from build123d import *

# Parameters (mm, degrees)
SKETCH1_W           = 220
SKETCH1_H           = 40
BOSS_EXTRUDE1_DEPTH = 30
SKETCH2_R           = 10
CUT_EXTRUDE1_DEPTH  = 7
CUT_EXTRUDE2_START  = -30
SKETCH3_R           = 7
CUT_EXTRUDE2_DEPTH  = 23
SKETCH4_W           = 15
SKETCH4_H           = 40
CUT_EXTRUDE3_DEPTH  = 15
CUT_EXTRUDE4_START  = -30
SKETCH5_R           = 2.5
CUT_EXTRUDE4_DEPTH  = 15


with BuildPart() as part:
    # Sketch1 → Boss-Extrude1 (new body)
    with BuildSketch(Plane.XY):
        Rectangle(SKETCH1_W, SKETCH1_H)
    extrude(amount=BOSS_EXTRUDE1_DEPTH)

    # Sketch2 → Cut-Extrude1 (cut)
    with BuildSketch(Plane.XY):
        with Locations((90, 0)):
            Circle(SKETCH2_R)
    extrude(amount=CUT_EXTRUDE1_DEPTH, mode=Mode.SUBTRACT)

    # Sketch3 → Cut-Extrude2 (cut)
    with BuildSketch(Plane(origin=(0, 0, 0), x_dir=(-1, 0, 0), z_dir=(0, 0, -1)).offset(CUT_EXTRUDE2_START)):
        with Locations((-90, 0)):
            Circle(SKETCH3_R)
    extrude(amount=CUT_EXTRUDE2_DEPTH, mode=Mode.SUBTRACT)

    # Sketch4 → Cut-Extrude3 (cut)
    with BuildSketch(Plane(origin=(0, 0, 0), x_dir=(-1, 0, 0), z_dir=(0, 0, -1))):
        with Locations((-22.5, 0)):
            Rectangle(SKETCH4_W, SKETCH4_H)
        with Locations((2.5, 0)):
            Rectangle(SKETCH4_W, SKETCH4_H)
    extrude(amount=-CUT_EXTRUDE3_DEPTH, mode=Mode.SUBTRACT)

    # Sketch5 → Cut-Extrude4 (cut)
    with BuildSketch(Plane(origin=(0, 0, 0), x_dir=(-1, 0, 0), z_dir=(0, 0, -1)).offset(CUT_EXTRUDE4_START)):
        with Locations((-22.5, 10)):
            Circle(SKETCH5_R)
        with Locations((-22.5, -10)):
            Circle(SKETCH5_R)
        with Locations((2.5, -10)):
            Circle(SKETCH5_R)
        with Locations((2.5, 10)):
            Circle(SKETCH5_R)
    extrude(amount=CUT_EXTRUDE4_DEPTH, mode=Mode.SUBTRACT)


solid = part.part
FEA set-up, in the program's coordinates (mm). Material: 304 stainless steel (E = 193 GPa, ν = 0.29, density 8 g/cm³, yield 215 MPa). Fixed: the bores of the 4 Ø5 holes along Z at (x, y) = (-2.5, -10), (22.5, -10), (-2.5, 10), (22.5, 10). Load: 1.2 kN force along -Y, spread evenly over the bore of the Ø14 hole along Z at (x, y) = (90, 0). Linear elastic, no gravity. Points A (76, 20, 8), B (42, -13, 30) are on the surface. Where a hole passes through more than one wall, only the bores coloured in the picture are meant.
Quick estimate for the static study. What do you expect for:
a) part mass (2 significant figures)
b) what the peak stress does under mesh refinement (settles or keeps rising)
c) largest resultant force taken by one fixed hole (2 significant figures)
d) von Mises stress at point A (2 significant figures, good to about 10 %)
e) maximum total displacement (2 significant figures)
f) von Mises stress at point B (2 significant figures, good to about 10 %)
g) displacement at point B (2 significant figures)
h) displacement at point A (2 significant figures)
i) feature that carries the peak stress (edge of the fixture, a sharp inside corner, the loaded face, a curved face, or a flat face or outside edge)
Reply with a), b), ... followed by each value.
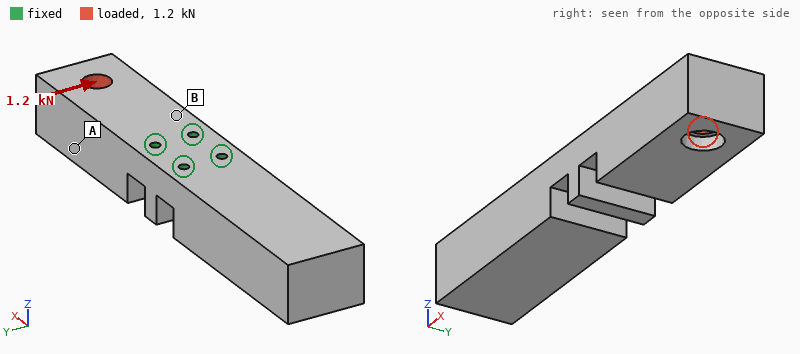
a) 1.9 kg
b) keeps rising
c) 2.9 kN
d) 2.5 MPa
e) 13 µm
f) 8.7 MPa
g) 2.3 µm
h) 7.3 µm
i) edge of the fixture
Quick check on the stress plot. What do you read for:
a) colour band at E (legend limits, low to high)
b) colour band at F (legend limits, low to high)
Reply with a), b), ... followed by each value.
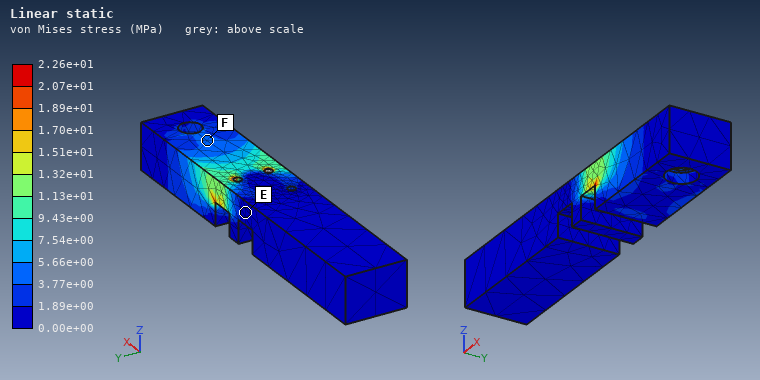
a) 0.00e+00 to 1.89e+00 MPa
b) 3.77e+00 to 5.66e+00 MPa
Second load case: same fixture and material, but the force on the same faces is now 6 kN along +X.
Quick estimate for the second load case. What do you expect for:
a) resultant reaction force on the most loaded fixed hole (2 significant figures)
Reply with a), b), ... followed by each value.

a) 2.7 kN
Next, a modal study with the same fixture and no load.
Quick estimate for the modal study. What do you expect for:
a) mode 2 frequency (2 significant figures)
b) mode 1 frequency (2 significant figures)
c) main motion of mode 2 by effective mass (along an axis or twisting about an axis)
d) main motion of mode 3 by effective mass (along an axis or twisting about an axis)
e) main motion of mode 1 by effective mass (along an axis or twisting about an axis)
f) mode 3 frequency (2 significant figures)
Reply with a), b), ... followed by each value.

a) 1400 Hz
b) 960 Hz
c) along Z
d) along Y
e) along Z
f) 1900 Hz
